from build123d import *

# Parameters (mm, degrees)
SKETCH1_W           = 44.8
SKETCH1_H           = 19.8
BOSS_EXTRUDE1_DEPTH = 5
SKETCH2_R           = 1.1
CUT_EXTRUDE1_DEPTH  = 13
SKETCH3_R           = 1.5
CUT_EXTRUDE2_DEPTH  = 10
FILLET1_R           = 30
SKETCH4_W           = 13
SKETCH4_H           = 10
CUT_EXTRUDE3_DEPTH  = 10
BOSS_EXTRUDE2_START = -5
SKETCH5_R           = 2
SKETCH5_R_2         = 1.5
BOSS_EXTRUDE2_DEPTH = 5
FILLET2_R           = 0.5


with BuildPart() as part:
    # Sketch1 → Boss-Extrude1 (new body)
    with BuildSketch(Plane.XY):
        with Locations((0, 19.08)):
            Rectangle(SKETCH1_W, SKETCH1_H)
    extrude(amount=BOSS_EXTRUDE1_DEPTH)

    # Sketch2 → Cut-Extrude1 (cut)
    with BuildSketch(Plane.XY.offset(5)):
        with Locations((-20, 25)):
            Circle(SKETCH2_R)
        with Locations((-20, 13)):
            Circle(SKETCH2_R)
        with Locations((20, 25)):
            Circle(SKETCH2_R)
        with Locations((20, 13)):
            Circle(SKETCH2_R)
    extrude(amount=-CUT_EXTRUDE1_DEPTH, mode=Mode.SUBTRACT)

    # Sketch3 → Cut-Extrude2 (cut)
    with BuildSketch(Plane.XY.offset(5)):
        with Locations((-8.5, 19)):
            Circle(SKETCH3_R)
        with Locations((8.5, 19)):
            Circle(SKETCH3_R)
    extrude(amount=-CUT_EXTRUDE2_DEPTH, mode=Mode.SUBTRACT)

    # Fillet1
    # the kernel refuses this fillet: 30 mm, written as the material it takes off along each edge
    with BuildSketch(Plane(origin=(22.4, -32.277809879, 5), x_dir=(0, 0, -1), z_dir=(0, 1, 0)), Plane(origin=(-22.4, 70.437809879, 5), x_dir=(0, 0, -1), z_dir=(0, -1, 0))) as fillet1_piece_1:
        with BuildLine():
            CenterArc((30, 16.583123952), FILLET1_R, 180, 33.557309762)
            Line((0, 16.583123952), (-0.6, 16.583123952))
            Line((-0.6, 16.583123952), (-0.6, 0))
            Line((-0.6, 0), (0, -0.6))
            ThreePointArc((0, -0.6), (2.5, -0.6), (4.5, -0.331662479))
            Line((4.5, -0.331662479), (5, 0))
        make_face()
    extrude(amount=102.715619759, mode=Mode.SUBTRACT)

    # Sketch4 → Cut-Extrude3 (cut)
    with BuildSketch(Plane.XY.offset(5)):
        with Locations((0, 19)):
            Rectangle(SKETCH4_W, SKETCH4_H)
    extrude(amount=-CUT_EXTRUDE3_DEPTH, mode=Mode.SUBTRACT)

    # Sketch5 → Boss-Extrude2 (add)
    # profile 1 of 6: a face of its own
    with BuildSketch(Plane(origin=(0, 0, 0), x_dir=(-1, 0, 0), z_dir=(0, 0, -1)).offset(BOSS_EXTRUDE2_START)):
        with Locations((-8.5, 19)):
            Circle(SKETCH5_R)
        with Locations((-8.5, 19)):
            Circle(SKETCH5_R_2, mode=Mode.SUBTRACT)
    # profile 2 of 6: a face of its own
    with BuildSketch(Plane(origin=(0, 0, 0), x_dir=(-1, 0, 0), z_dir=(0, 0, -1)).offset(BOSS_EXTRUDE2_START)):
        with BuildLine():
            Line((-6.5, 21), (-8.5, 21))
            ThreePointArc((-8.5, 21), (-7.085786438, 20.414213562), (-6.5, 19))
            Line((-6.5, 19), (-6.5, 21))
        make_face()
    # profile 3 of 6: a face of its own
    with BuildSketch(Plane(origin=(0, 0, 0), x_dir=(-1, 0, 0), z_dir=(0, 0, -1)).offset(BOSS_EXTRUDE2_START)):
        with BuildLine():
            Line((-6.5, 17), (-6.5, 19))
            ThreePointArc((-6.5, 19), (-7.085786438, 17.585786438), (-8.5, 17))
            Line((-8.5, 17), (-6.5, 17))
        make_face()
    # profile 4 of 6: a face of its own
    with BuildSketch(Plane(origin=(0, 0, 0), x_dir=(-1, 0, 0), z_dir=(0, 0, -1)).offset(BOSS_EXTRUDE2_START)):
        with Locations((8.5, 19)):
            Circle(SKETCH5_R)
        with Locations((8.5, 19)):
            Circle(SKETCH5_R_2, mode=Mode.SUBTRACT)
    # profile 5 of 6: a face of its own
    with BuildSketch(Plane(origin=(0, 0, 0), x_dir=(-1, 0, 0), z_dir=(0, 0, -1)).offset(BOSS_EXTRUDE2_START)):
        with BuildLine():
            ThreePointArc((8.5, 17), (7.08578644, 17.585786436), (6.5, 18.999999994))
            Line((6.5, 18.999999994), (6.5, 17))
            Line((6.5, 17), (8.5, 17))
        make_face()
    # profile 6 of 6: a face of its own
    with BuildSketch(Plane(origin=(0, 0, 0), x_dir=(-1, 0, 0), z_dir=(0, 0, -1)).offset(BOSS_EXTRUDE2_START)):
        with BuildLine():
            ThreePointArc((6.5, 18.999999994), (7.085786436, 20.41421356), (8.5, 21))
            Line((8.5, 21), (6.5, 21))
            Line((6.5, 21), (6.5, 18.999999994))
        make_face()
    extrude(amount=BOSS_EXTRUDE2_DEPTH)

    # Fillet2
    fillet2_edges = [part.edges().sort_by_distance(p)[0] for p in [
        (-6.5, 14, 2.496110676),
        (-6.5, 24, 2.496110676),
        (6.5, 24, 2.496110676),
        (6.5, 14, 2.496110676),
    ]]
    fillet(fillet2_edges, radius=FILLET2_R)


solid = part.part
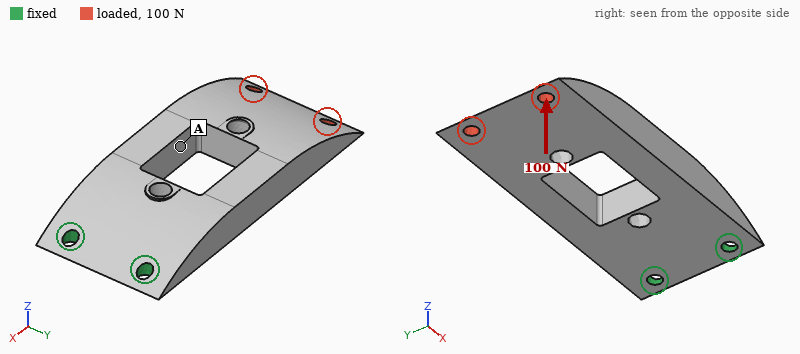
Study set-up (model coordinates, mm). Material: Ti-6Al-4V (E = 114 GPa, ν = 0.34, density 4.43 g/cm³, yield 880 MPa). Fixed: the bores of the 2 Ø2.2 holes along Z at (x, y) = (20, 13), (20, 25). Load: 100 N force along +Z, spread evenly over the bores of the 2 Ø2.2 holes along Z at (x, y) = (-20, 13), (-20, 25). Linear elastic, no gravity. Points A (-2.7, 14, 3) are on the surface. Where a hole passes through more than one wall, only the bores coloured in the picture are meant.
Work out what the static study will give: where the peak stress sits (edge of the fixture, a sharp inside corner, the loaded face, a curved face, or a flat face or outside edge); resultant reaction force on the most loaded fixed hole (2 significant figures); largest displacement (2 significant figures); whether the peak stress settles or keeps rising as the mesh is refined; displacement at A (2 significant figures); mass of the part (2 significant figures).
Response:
edge of the fixture
51 N
0.49 mm
keeps rising
0.22 mm
12 g
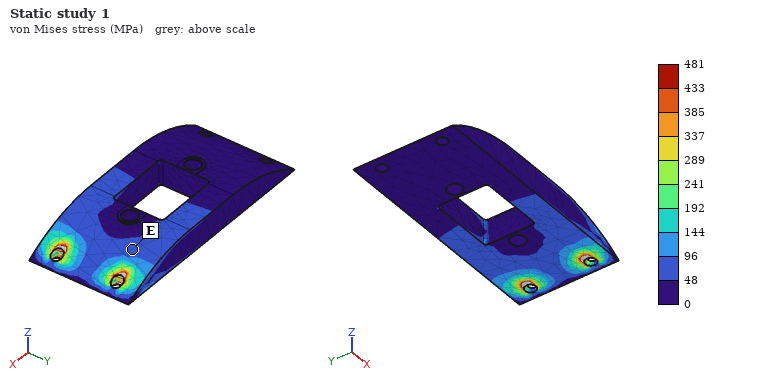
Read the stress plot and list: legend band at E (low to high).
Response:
48 to 96 MPa
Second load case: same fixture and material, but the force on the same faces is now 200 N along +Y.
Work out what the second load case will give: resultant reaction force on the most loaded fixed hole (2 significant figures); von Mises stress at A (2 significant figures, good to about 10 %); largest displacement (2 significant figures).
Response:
620 N
22 MPa
48 µm
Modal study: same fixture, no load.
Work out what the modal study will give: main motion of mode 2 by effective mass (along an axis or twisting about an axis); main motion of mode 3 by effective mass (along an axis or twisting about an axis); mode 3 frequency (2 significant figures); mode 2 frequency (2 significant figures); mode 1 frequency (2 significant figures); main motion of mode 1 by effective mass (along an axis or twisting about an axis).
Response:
along Y
along Y
7000 Hz
5500 Hz
1300 Hz
along Z
